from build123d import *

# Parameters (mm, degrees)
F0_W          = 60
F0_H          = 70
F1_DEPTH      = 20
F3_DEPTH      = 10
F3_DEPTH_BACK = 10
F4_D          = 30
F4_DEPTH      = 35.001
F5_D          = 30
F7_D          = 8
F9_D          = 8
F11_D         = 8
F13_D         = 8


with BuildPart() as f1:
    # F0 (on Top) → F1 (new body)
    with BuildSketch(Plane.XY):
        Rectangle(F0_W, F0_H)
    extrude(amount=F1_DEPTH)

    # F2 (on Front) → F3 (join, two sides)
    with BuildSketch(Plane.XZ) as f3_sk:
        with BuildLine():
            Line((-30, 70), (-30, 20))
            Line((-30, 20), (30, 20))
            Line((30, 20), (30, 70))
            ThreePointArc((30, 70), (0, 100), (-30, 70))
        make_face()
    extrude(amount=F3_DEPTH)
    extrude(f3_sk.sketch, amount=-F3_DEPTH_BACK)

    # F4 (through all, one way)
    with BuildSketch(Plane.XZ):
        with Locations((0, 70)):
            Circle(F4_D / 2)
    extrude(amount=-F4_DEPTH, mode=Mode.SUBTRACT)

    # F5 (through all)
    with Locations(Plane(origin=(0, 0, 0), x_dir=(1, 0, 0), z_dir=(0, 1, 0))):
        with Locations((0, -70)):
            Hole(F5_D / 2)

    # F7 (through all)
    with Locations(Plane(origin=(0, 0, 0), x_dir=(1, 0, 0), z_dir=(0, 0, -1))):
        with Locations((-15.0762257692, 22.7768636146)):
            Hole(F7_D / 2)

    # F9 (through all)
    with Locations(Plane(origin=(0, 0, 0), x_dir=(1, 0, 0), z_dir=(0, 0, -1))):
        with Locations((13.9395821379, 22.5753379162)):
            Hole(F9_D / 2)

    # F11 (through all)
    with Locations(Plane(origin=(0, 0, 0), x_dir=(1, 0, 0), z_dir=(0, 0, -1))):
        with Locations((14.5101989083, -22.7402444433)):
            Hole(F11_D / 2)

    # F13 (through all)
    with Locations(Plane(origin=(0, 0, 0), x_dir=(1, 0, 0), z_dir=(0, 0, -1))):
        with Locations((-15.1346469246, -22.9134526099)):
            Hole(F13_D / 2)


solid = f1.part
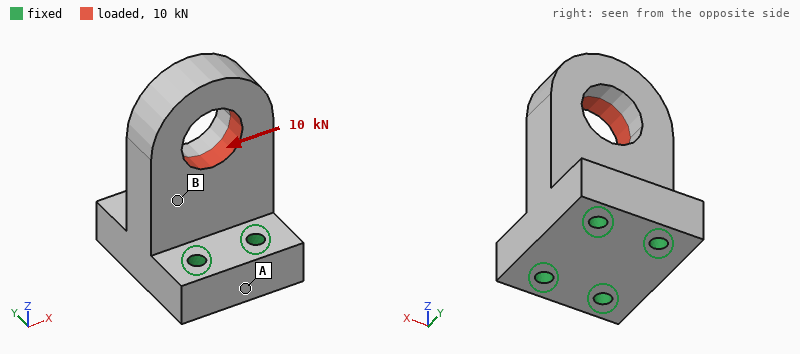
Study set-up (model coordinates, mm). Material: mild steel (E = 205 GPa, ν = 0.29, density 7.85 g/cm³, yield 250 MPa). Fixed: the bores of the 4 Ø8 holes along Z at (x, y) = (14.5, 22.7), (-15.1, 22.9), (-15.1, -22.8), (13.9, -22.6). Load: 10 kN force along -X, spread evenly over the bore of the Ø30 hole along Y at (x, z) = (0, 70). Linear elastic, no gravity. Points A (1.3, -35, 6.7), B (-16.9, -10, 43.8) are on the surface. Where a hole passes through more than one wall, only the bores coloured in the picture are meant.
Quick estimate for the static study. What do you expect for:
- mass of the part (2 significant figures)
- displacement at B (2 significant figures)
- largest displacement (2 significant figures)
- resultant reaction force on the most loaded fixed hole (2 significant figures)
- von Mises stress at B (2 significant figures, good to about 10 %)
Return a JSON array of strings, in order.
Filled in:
["1.2 kg", "16 µm", "51 µm", "7.8 kN", "20 MPa"]
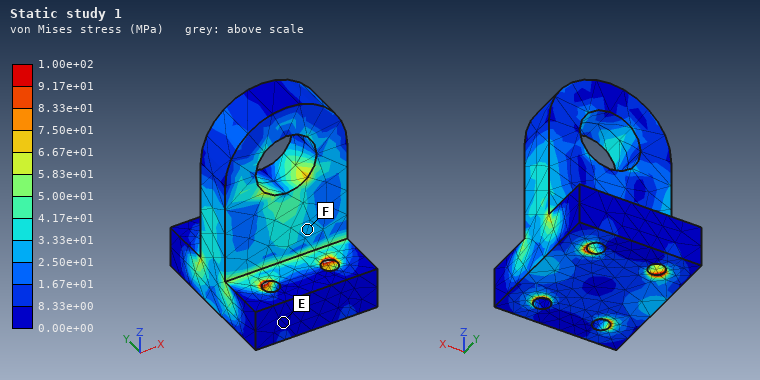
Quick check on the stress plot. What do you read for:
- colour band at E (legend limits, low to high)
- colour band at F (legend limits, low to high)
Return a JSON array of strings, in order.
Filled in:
["0.00e+00 to 8.33e+00 MPa", "2.50e+01 to 3.33e+01 MPa"]
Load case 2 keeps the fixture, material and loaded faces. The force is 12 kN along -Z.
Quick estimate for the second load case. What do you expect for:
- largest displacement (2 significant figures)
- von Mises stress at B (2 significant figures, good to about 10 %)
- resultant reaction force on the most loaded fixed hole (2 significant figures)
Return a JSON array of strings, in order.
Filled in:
["31 µm", "27 MPa", "3.9 kN"]
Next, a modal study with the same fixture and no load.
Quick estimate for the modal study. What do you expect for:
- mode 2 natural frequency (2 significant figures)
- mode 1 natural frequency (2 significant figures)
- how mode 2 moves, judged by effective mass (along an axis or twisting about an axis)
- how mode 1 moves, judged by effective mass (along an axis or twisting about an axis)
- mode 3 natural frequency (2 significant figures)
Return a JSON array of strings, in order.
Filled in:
["4300 Hz", "2600 Hz", "along X", "along Y", "6400 Hz"]
